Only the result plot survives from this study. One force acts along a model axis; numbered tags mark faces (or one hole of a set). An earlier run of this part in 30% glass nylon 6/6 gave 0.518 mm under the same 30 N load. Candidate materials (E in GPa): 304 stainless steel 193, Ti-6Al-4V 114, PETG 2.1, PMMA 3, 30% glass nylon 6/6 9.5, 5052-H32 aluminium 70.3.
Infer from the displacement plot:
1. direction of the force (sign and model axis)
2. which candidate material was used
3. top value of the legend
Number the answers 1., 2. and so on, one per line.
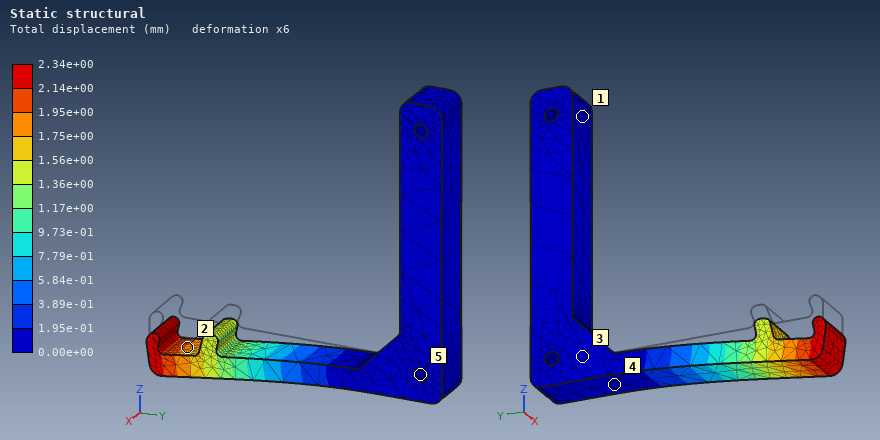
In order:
1. -Z
2. PETG
3. 2.34e+00 mm
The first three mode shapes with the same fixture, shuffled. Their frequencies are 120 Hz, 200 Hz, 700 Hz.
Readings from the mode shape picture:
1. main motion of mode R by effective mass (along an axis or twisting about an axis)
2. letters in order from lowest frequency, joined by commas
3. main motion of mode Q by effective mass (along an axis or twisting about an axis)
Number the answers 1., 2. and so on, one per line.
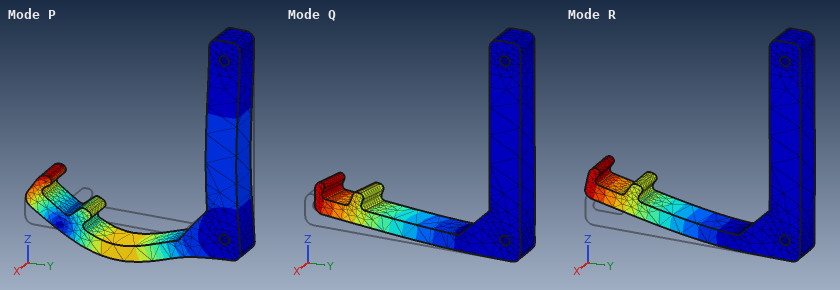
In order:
1. along Z
2. R, Q, P
3. along X
